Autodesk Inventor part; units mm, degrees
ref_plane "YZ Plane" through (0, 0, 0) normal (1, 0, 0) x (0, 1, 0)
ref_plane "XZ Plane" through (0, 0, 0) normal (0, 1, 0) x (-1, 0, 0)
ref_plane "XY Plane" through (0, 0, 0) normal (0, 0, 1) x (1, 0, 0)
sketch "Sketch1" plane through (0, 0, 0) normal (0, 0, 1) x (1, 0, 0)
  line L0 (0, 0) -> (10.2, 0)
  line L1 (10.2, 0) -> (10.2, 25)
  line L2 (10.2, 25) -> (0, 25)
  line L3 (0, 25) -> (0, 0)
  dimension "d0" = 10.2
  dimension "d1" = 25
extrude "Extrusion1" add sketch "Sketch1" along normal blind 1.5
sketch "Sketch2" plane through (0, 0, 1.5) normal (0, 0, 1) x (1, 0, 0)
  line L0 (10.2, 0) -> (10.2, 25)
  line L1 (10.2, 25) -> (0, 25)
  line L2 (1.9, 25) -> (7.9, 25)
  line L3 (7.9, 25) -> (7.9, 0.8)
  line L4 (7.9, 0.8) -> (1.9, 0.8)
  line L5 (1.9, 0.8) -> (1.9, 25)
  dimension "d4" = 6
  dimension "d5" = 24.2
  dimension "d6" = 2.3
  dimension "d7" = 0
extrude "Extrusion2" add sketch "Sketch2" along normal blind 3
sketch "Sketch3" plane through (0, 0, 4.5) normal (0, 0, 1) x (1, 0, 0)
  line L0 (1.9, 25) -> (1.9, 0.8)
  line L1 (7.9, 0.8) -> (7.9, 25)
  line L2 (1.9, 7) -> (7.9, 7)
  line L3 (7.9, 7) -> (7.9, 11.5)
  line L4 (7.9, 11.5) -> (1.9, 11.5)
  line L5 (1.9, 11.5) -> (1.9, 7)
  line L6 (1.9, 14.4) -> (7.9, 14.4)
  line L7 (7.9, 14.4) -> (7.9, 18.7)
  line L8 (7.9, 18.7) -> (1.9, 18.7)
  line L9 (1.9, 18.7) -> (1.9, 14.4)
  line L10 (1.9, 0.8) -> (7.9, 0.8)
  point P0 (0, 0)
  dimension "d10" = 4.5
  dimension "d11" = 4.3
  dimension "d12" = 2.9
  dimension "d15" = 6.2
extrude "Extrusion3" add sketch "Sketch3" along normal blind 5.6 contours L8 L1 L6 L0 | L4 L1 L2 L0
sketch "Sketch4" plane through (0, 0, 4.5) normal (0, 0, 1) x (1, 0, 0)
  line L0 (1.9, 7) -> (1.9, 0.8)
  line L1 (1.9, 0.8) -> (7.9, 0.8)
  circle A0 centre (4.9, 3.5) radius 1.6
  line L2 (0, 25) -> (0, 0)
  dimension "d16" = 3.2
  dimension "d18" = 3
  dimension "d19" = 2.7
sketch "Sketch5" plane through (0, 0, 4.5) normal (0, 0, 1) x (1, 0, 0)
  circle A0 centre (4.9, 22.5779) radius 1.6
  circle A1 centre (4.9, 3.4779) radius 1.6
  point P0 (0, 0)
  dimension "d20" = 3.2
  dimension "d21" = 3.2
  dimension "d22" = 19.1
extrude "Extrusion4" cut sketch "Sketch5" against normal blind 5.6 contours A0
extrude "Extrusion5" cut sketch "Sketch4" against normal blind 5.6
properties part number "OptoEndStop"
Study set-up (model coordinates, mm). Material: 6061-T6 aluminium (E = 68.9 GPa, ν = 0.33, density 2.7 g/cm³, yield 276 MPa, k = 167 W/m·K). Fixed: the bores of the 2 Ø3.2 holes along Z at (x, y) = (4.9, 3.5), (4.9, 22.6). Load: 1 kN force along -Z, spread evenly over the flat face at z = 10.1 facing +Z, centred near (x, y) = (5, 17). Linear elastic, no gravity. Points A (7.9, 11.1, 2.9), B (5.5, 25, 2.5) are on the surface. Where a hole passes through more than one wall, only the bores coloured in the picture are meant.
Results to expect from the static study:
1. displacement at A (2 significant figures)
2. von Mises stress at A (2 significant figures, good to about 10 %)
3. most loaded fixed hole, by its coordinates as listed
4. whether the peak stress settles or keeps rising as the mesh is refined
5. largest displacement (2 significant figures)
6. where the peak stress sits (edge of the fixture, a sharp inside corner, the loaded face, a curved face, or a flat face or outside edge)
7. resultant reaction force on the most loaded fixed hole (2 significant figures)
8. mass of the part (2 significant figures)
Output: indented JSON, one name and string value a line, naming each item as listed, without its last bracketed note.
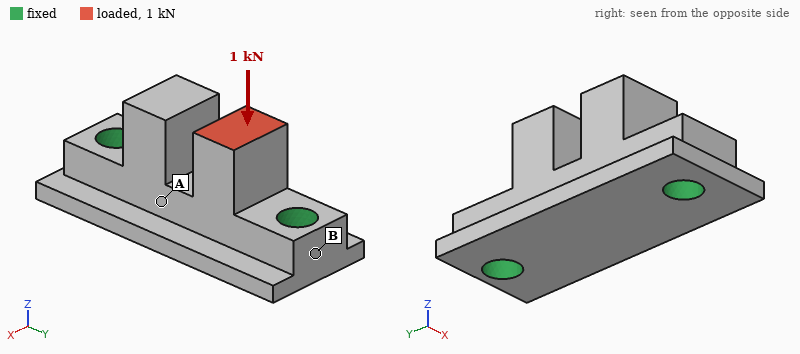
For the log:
{
  "displacement at A": "6.5 µm",
  "von Mises stress at A": "29 MPa",
  "most loaded fixed hole, by its coordinates as listed": "(4.9, 22.6)",
  "whether the peak stress settles or keeps rising as the mesh is refined": "keeps rising",
  "largest displacement": "15 µm",
  "where the peak stress sits": "edge of the fixture",
  "resultant reaction force on the most loaded fixed hole": "750 N",
  "mass of the part": "2.8 g"
}
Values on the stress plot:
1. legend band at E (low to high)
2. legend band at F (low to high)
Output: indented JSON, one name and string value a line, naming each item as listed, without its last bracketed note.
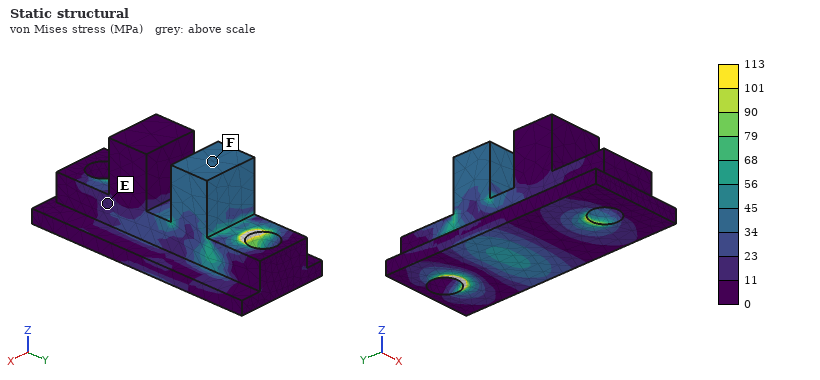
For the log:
{
  "legend band at E": "11 to 23 MPa",
  "legend band at F": "34 to 45 MPa"
}
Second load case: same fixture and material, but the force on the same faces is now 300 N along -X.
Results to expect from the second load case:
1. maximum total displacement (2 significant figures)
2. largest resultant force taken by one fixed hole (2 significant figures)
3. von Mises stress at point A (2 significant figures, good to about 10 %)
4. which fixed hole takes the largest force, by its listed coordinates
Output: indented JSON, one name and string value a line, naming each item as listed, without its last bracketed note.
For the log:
{
  "maximum total displacement": "30 µm",
  "largest resultant force taken by one fixed hole": "230 N",
  "von Mises stress at point A": "34 MPa",
  "which fixed hole takes the largest force, by its listed coordinates": "(4.9, 22.6)"
}
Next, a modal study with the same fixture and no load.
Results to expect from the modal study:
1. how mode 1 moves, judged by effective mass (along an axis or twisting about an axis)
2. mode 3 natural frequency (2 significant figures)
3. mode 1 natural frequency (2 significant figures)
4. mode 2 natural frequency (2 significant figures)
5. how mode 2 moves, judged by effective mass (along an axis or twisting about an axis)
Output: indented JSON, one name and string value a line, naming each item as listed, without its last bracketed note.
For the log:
{
  "how mode 1 moves, judged by effective mass": "along X",
  "mode 3 natural frequency": "47 kHz",
  "mode 1 natural frequency": "30 kHz",
  "mode 2 natural frequency": "37 kHz",
  "how mode 2 moves, judged by effective mass": "along Z"
}
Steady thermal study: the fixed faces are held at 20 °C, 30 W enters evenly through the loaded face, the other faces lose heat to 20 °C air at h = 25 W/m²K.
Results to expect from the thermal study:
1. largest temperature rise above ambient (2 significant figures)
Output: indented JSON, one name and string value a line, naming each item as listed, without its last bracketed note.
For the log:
{
  "largest temperature rise above ambient": "63 K"
}
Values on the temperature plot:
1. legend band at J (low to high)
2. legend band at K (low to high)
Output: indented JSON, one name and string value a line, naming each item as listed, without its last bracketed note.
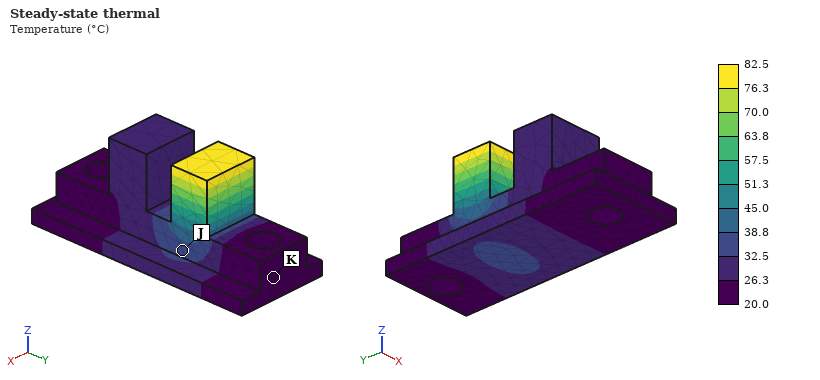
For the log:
{
  "legend band at J": "32.5 to 38.8 °C",
  "legend band at K": "20.0 to 26.3 °C"
}
